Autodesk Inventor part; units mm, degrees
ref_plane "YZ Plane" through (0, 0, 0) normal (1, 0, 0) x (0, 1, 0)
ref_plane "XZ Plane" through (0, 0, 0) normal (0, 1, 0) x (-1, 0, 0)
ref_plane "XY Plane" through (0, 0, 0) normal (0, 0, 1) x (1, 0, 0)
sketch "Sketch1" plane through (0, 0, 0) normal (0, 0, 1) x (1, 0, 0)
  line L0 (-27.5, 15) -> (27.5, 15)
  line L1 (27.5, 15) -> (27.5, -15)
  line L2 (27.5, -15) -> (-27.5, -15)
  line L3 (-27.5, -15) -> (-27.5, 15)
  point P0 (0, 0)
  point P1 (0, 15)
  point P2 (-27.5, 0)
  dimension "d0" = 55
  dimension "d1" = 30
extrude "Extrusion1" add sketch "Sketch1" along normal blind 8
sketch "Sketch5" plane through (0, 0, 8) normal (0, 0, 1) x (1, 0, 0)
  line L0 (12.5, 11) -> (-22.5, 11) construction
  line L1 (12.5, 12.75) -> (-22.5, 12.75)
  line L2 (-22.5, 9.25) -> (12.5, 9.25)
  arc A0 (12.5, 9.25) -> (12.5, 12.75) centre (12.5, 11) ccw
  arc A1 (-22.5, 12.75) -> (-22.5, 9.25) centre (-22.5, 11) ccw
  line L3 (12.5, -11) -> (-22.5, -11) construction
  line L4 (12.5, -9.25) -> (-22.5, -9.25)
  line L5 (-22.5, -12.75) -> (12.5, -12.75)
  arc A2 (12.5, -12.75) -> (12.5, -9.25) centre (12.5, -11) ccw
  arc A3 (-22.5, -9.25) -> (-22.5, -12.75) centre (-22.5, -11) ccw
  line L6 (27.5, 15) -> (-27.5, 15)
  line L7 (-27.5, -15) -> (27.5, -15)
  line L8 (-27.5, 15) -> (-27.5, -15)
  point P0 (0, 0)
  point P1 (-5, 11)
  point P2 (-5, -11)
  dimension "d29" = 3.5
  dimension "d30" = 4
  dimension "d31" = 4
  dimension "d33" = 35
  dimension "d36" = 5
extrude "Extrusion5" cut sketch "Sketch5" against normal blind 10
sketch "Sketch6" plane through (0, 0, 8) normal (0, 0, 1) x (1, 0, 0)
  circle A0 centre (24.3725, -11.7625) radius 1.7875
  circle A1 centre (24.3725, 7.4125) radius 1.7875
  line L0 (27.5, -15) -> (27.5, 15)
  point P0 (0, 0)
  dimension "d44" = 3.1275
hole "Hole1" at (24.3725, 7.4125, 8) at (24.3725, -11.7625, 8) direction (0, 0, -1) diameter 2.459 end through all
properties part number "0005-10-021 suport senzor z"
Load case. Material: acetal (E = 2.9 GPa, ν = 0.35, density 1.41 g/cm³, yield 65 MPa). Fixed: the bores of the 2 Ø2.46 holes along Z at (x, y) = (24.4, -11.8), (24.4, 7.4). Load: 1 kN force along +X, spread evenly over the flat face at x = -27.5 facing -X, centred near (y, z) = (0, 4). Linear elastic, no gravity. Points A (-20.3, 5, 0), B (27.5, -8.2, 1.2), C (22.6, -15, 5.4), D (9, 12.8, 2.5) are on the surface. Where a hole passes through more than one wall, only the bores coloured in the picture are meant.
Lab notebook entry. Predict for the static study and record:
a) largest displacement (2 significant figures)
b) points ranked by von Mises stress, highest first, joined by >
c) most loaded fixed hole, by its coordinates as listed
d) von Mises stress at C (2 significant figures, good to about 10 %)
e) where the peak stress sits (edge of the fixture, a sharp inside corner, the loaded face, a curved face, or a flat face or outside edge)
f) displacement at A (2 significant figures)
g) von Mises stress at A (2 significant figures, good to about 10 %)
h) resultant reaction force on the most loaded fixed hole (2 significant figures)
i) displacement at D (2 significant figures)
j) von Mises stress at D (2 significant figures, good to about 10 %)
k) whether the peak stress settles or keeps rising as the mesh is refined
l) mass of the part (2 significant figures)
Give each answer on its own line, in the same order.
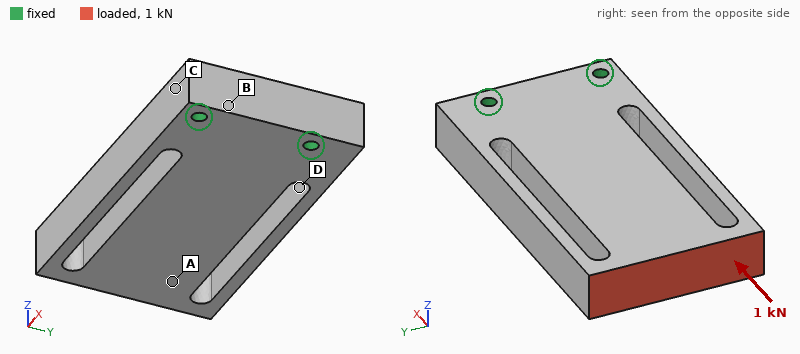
0.12 mm
D > A > C > B
(24.4, 7.4)
2.7 MPa
edge of the fixture
0.089 mm
4.7 MPa
610 N
0.049 mm
6.9 MPa
keeps rising
16 g
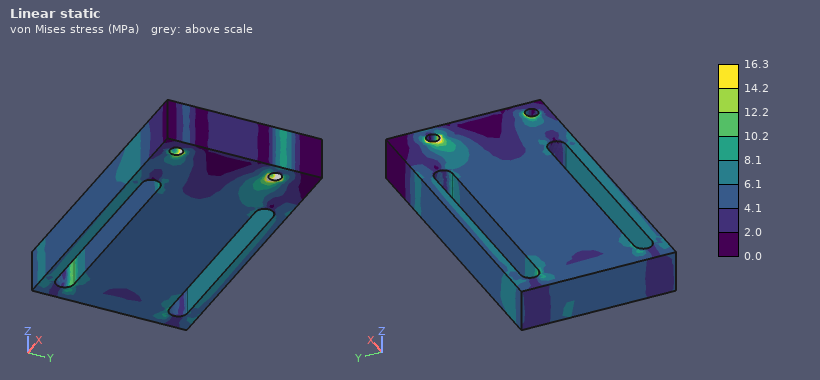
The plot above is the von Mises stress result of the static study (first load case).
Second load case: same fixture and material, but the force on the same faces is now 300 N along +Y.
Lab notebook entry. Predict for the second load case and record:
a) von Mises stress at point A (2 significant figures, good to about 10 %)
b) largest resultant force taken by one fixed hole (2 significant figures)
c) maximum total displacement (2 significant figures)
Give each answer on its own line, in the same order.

4.7 MPa
810 N
0.69 mm
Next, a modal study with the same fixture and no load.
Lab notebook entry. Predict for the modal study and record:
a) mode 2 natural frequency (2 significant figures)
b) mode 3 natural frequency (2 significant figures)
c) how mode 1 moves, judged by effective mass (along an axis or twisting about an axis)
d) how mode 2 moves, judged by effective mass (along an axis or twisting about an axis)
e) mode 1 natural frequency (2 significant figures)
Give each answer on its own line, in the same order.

1500 Hz
2100 Hz
along Z
along Y
630 Hz
